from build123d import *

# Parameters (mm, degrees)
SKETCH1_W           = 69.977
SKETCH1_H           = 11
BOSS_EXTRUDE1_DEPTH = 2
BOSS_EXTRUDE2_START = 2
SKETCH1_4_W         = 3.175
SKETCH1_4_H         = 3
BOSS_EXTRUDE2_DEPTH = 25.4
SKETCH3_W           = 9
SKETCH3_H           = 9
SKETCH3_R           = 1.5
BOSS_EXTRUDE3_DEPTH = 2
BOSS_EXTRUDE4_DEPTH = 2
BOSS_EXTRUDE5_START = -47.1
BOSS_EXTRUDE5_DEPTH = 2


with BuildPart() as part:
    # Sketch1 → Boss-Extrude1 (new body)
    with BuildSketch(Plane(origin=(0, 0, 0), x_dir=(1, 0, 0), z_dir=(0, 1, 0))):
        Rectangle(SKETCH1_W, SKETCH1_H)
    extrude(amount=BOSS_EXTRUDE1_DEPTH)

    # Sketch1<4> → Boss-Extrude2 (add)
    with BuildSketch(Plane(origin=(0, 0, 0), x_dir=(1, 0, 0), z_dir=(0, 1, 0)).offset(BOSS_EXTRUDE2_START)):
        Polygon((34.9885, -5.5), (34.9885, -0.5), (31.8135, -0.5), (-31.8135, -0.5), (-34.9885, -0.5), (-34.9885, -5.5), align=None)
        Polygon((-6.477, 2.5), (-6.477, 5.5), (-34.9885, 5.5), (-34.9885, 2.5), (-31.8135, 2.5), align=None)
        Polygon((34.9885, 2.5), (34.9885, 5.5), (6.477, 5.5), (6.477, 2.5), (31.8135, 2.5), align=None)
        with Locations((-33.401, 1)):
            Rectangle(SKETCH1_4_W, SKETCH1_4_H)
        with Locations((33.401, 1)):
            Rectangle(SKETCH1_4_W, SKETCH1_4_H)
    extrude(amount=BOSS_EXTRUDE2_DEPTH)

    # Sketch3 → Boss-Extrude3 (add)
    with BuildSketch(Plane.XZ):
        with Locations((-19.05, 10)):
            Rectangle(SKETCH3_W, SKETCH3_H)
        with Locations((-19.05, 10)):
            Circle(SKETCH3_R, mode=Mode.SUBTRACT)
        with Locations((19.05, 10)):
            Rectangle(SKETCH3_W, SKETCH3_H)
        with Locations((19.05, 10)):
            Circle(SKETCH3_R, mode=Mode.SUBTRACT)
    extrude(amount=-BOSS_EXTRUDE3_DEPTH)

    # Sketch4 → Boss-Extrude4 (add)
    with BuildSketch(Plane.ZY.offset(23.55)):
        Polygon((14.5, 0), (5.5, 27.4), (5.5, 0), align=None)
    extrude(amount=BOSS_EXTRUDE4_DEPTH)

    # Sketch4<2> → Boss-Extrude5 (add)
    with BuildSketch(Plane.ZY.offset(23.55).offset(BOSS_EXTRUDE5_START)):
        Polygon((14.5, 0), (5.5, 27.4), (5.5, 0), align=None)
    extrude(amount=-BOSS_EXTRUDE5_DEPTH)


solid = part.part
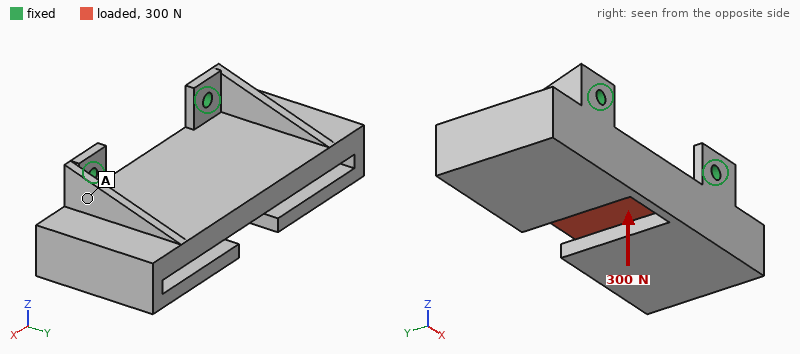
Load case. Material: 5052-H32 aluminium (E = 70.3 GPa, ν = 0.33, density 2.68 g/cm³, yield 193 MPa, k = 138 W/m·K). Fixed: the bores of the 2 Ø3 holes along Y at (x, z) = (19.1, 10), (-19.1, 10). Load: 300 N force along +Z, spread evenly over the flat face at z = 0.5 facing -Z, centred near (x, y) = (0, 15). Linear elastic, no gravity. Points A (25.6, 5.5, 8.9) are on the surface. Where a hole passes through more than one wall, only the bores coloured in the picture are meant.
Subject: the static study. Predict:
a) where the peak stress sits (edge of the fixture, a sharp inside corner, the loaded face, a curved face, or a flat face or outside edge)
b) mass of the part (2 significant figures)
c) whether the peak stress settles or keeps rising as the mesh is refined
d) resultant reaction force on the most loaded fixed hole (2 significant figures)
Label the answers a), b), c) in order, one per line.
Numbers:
a) edge of the fixture
b) 43 g
c) keeps rising
d) 150 N
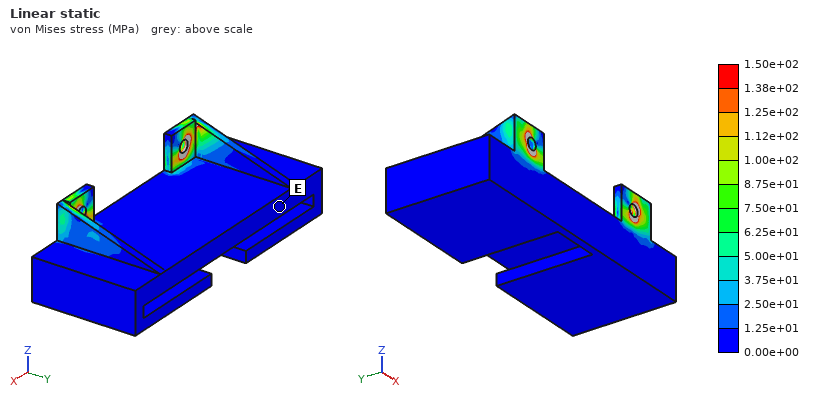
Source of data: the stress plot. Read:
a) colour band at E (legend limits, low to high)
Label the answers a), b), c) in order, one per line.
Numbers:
a) 0.00e+00 to 1.25e+01 MPa
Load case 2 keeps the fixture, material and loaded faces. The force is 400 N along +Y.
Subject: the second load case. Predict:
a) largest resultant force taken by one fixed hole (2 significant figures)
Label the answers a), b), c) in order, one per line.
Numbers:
a) 200 N
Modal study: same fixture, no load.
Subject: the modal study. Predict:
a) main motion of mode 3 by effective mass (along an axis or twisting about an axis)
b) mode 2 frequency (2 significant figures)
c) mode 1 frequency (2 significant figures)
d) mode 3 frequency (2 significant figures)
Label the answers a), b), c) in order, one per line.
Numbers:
a) along X
b) 2800 Hz
c) 1100 Hz
d) 5000 Hz
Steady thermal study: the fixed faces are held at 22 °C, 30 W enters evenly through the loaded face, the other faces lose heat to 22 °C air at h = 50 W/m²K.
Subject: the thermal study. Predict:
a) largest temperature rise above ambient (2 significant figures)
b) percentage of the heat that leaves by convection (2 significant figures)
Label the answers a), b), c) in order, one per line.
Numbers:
a) 27 K
b) 27 %
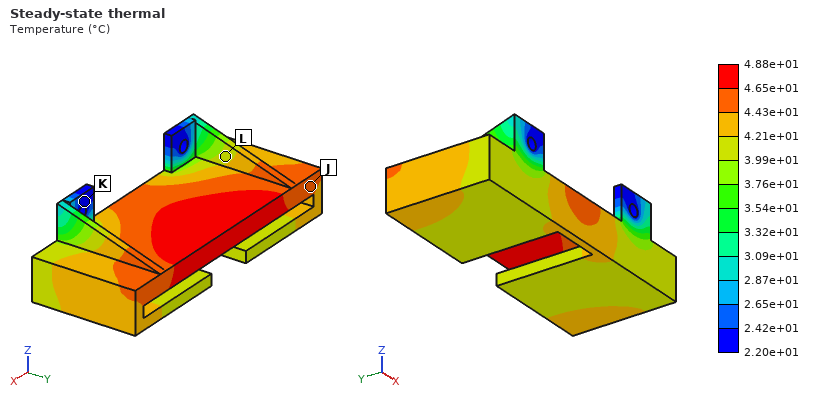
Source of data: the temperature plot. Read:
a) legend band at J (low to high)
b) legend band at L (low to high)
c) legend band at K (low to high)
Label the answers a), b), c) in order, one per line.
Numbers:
a) 4.43e+01 to 4.65e+01 °C
b) 3.99e+01 to 4.21e+01 °C
c) 2.20e+01 to 2.42e+01 °C
